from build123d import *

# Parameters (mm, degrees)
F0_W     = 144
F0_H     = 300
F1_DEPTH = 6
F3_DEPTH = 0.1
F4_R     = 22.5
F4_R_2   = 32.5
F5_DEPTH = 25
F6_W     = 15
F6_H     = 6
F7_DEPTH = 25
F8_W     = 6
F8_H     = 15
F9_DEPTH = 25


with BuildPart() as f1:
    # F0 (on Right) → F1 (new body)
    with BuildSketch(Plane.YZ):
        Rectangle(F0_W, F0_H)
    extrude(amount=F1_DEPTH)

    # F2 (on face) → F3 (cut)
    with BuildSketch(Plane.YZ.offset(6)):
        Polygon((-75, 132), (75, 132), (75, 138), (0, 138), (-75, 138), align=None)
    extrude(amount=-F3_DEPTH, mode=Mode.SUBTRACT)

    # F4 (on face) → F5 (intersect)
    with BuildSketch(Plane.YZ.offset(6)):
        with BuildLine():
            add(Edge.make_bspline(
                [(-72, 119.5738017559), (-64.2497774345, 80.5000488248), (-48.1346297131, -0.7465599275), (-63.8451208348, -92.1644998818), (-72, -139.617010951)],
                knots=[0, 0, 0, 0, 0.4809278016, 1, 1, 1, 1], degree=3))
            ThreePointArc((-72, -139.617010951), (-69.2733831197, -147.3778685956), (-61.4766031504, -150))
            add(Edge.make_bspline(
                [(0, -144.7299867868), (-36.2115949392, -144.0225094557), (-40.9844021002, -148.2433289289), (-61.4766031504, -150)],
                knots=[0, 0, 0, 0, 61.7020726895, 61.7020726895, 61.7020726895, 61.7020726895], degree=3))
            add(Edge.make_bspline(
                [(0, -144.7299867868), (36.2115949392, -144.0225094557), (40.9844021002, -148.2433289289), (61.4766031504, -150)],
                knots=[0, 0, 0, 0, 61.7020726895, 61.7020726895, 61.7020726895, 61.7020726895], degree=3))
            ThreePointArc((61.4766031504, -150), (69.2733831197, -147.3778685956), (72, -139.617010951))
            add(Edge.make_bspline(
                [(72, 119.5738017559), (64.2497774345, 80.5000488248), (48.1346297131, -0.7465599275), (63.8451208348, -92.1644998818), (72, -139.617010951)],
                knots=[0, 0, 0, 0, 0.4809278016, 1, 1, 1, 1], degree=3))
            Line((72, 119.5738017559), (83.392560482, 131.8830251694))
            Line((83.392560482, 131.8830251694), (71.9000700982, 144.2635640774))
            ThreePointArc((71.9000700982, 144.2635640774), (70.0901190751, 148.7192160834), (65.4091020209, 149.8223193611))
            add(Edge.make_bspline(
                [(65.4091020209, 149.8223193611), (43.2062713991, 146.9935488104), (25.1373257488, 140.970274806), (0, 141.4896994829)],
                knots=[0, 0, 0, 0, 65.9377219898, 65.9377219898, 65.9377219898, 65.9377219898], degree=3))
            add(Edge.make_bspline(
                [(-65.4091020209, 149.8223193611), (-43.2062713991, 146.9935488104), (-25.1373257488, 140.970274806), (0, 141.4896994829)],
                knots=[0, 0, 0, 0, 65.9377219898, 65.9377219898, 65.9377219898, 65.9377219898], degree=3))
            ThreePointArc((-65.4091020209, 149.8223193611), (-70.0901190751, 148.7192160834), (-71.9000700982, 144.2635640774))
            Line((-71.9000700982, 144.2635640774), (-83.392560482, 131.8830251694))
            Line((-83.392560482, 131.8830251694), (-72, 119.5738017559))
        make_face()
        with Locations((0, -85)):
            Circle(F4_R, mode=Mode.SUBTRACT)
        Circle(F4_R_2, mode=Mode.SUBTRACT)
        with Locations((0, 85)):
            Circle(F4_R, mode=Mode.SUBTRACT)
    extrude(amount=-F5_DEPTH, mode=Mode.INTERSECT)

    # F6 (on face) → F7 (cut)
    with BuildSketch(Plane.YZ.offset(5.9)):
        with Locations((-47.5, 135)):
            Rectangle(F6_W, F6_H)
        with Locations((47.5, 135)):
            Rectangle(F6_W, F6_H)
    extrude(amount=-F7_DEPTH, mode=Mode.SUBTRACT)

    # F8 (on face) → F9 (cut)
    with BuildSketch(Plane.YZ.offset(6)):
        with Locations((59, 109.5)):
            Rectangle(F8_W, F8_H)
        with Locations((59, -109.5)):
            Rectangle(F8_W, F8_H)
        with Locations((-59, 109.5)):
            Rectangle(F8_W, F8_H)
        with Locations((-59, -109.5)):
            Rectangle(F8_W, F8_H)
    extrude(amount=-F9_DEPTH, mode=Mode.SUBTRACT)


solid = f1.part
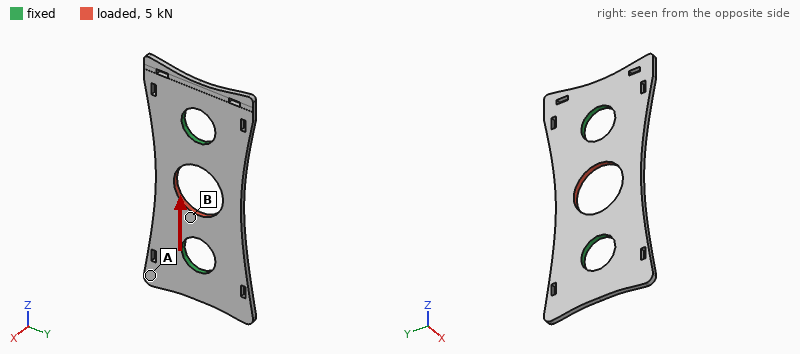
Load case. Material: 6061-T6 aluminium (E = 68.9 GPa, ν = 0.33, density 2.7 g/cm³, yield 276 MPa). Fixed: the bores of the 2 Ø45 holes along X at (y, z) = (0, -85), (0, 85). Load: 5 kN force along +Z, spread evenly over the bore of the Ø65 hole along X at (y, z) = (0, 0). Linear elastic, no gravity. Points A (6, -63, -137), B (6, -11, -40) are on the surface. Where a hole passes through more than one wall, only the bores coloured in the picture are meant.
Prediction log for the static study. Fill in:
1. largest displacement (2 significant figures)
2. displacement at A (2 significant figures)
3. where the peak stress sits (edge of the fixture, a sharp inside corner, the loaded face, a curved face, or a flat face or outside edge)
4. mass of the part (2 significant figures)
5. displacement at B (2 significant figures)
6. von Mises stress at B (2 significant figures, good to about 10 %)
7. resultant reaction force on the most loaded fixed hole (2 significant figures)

5.2 µm
1.5 µm
the loaded face
480 g
2.1 µm
5.8 MPa
2.5 kN
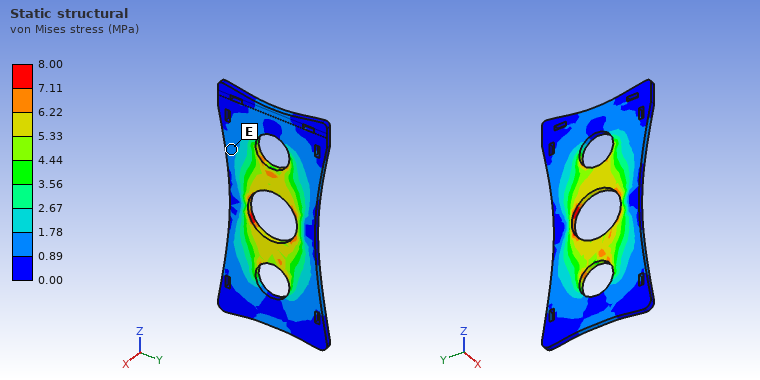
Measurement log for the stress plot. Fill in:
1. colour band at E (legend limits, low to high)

0.89 to 1.78 MPa
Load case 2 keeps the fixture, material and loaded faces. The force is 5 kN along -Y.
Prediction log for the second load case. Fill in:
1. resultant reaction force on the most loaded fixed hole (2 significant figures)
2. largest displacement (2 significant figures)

2.5 kN
14 µm
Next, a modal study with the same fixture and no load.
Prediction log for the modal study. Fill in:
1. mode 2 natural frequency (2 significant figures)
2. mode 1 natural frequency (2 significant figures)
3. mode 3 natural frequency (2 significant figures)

1500 Hz
1400 Hz
1500 Hz
